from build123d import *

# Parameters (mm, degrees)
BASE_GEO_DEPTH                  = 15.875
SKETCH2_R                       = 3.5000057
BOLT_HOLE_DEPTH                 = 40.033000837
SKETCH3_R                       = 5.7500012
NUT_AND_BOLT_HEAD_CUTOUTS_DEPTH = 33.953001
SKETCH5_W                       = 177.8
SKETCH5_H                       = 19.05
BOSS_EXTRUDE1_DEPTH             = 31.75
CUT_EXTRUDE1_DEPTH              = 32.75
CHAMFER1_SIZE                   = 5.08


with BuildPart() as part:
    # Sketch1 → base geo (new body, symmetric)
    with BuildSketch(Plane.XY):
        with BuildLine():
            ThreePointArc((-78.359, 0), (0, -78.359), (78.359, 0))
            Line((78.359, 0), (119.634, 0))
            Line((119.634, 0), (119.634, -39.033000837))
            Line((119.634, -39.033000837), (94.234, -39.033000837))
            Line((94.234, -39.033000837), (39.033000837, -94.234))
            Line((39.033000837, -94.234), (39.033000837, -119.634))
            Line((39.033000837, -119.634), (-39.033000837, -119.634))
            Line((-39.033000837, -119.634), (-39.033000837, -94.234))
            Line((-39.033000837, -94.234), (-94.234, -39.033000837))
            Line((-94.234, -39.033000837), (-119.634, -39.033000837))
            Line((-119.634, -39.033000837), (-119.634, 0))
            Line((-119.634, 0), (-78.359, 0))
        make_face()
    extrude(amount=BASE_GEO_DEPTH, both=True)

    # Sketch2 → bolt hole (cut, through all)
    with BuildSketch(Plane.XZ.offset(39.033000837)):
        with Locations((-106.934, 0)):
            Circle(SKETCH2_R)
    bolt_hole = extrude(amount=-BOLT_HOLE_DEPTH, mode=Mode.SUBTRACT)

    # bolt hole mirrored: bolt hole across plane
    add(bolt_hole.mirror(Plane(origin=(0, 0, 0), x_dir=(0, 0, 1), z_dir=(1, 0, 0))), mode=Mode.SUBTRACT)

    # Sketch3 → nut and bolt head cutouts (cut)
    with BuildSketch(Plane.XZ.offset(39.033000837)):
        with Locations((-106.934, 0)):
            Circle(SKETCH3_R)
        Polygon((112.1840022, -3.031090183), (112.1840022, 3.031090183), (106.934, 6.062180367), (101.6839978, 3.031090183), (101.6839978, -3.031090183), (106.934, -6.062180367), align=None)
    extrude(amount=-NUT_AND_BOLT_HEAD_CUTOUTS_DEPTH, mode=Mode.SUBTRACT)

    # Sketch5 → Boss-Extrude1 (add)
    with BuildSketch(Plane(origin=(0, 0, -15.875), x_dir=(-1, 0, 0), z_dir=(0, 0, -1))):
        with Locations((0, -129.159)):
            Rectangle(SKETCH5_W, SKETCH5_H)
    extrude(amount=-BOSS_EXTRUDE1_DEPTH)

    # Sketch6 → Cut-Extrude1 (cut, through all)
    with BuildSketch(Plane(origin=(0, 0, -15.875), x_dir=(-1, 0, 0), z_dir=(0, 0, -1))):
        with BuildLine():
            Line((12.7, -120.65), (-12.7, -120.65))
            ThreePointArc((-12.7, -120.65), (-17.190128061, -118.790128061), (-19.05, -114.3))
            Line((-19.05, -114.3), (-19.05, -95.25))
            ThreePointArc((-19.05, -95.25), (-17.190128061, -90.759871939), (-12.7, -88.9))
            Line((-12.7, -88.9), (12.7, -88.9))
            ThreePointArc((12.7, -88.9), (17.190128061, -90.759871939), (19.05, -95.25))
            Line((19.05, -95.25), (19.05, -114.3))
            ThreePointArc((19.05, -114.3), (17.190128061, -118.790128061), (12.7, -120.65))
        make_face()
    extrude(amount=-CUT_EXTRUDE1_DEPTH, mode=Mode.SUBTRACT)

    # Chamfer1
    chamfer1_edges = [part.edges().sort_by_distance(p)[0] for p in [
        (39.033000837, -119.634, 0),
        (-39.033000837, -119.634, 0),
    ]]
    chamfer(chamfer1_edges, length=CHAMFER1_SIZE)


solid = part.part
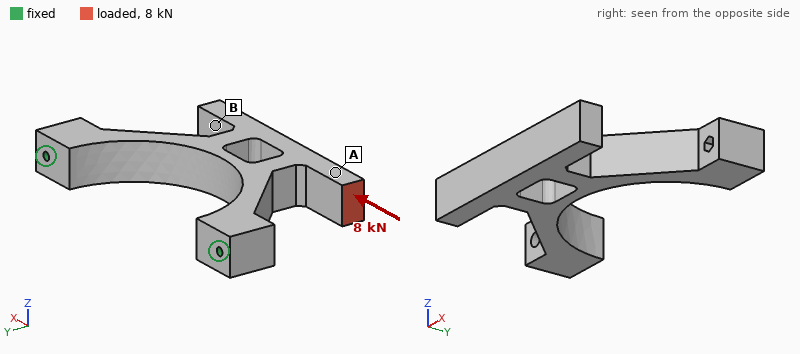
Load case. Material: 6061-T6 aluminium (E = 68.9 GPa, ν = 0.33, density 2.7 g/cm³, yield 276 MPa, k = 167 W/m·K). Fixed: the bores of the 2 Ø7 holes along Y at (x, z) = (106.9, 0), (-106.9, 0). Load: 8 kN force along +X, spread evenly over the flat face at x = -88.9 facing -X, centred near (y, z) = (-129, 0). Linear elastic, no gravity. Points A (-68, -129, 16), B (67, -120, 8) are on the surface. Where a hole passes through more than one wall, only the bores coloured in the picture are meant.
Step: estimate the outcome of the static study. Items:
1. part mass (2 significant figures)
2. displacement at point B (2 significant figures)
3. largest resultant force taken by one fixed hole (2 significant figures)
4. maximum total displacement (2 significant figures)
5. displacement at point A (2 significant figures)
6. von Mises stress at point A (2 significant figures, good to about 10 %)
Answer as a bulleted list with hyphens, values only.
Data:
- 950 g
- 66 µm
- 6.2 kN
- 92 µm
- 82 µm
- 13 MPa
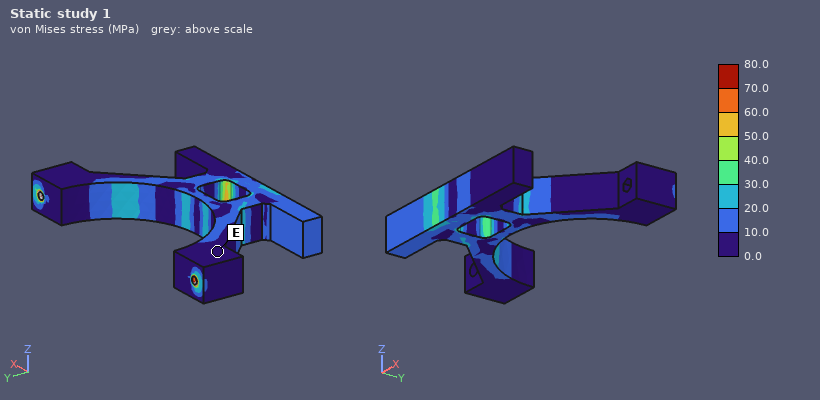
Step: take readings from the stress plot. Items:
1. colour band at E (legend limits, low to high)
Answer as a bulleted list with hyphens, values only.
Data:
- 0.0 to 10.0 MPa
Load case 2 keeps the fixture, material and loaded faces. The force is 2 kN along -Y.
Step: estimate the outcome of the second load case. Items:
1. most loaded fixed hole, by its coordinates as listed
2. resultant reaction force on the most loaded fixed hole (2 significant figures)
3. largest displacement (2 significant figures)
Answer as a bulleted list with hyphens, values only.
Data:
- (-106.9, 0)
- 2.2 kN
- 0.26 mm
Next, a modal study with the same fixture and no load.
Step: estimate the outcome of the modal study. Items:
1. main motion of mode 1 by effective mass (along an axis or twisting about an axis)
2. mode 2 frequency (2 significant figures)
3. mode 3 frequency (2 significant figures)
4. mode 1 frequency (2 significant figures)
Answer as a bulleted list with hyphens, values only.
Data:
- along Z
- 1200 Hz
- 1200 Hz
- 270 Hz
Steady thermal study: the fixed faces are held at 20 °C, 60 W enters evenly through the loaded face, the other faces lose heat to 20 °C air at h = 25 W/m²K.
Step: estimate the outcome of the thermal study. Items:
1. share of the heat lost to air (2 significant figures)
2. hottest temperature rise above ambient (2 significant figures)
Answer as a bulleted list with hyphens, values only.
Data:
- 45 %
- 65 K
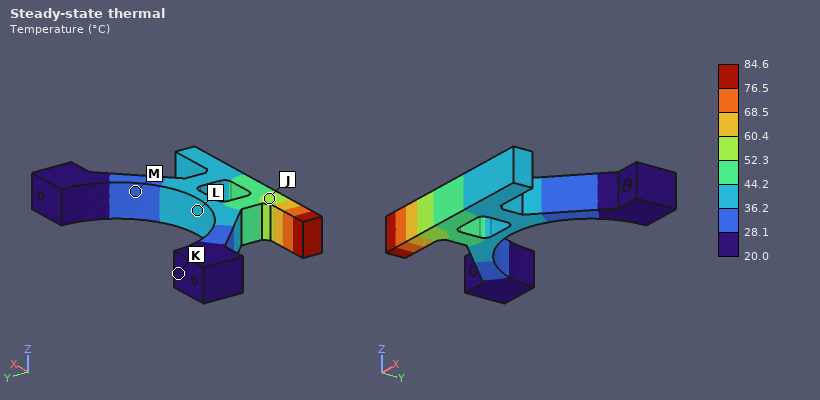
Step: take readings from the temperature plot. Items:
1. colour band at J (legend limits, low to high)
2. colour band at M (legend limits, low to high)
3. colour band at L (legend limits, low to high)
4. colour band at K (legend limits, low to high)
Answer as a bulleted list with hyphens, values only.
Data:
- 52.3 to 60.4 °C
- 28.1 to 36.2 °C
- 36.2 to 44.2 °C
- 20.0 to 28.1 °C
